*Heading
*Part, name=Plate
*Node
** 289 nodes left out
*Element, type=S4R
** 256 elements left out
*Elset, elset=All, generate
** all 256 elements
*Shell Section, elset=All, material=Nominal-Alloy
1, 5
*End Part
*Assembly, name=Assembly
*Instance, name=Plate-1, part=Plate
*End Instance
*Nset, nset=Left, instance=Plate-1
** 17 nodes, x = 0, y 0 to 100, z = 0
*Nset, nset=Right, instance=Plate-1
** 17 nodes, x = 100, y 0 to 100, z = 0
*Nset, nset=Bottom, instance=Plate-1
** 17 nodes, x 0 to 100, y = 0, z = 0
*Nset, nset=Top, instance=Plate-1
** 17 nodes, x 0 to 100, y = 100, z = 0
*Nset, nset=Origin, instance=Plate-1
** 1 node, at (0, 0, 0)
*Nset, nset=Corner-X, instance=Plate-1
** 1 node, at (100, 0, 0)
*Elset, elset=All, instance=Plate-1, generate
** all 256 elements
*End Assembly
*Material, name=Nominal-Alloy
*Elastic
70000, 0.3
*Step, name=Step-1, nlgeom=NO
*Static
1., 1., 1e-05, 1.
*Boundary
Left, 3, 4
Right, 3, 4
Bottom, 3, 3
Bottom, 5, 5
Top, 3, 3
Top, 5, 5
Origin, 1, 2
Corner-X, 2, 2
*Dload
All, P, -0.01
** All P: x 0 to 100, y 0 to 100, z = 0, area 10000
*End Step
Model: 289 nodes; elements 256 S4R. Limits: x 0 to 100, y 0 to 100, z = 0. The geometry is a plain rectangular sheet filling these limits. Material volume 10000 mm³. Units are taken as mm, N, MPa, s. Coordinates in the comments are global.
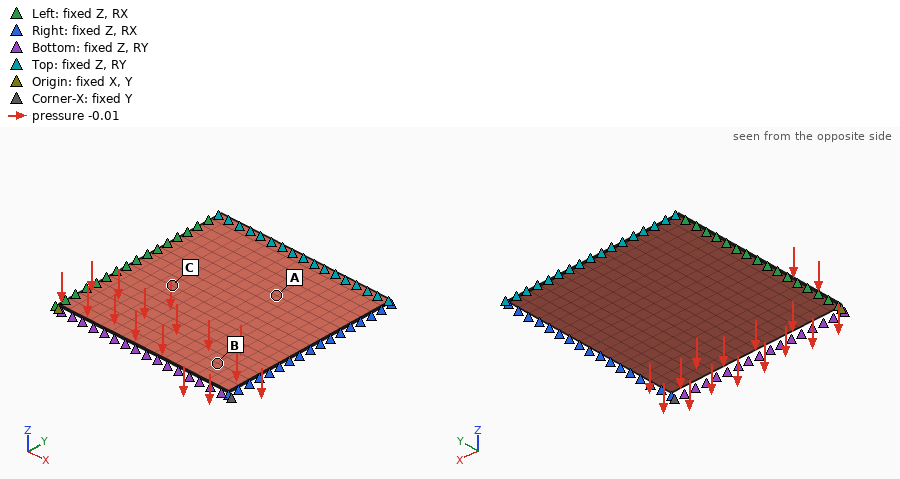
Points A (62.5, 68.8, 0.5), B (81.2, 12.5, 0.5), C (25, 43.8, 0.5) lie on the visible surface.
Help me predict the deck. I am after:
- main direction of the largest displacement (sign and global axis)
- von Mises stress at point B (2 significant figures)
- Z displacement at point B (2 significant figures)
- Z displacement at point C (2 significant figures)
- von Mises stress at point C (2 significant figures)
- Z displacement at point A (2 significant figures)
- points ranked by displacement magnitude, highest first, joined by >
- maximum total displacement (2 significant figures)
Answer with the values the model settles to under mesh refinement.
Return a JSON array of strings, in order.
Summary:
["-Z", "25 MPa", "-0.15 mm", "-0.45 mm", "22 MPa", "-0.50 mm", "A > C > B", "0.63 mm"]
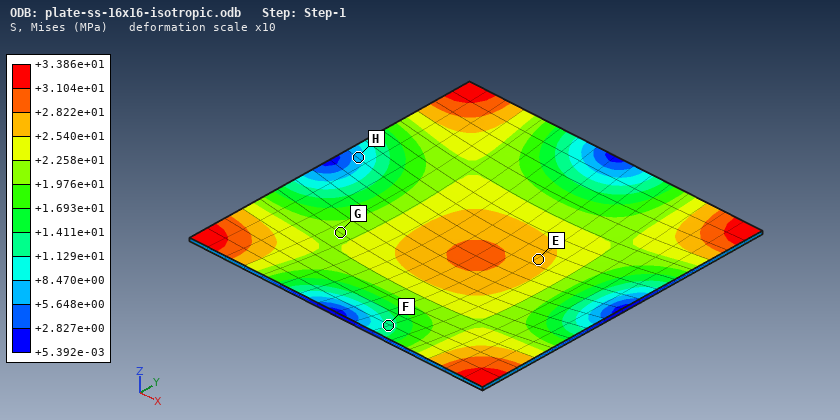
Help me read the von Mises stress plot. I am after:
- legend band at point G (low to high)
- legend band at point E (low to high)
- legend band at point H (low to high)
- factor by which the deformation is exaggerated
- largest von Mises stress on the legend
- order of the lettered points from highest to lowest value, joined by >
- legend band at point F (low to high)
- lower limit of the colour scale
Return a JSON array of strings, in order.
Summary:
["+1.976e+01 to +2.258e+01 MPa", "+2.540e+01 to +2.822e+01 MPa", "+5.648e+00 to +8.470e+00 MPa", "10", "+3.386e+01 MPa", "E > G > F > H", "+1.129e+01 to +1.411e+01 MPa", "+5.392e-03 MPa"]
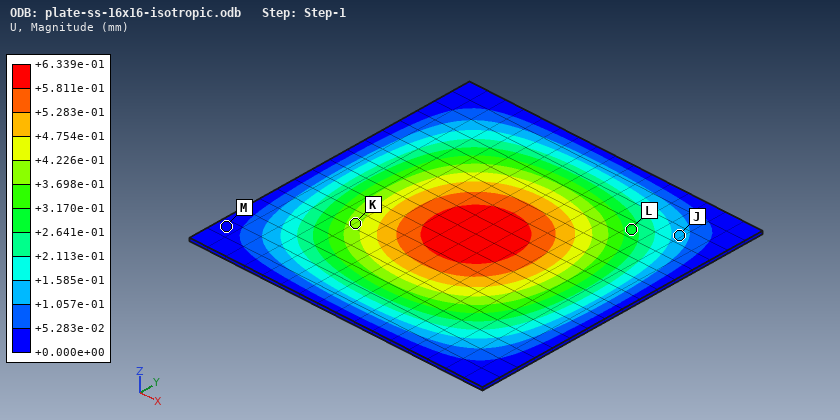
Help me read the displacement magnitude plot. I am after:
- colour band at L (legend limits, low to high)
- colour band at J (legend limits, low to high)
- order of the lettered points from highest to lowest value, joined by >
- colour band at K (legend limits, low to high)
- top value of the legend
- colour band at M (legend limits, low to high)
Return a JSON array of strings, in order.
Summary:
["+2.641e-01 to +3.170e-01 mm", "+1.057e-01 to +1.585e-01 mm", "K > L > J > M", "+3.698e-01 to +4.226e-01 mm", "+6.339e-01 mm", "+0.000e+00 to +5.283e-02 mm"]
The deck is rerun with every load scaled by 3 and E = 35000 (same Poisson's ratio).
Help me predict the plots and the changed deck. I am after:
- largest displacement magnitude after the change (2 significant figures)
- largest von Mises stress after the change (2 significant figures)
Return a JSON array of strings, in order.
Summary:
["3.8 mm", "100 MPa"]
